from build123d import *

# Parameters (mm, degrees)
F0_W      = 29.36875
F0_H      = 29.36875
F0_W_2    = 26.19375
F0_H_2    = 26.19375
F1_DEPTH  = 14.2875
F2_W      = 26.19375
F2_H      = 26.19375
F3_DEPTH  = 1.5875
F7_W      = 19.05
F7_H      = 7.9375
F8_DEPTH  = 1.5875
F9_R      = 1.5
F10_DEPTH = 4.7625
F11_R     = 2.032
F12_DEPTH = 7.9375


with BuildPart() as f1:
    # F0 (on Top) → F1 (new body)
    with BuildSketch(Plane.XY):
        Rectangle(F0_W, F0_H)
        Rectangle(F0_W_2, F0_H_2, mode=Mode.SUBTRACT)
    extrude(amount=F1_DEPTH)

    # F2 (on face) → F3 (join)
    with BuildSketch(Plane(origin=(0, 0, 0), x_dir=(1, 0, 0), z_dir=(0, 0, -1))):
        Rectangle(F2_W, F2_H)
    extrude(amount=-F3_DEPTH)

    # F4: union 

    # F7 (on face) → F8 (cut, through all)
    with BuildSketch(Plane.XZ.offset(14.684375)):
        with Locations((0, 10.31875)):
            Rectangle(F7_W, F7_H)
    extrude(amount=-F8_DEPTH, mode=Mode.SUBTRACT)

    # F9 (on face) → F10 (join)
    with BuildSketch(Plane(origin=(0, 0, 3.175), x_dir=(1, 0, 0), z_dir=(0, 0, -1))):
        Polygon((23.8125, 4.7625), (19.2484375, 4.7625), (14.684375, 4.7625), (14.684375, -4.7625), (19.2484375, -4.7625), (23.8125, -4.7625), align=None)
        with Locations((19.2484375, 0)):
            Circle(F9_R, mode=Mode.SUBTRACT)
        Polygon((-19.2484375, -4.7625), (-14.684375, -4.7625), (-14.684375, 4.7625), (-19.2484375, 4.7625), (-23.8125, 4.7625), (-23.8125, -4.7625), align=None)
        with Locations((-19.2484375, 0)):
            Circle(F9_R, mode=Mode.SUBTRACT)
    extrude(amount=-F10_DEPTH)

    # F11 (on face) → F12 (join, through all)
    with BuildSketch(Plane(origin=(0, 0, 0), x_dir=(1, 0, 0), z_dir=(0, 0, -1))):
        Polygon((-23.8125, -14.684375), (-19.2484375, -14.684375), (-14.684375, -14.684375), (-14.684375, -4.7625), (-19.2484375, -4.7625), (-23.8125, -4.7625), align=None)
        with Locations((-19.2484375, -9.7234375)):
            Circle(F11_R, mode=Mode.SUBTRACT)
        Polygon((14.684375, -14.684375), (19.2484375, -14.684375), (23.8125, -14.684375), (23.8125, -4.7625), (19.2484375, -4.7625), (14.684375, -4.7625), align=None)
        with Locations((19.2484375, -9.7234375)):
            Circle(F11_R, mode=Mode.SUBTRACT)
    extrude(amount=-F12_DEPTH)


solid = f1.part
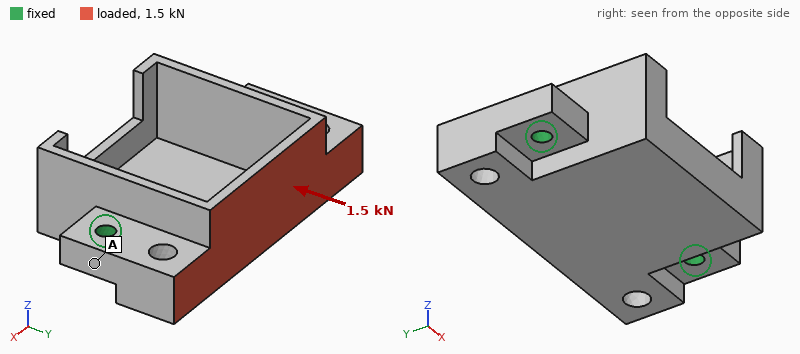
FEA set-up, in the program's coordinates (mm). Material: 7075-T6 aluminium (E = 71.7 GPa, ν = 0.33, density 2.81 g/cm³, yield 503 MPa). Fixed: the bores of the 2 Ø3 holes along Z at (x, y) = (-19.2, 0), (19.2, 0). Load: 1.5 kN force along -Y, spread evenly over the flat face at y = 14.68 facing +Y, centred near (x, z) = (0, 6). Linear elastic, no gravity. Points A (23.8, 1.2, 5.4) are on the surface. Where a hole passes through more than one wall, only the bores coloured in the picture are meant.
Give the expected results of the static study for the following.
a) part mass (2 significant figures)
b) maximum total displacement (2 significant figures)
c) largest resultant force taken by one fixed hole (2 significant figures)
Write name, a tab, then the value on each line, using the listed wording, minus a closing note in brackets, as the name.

part mass	15 g
maximum total displacement	0.18 mm
largest resultant force taken by one fixed hole	780 N
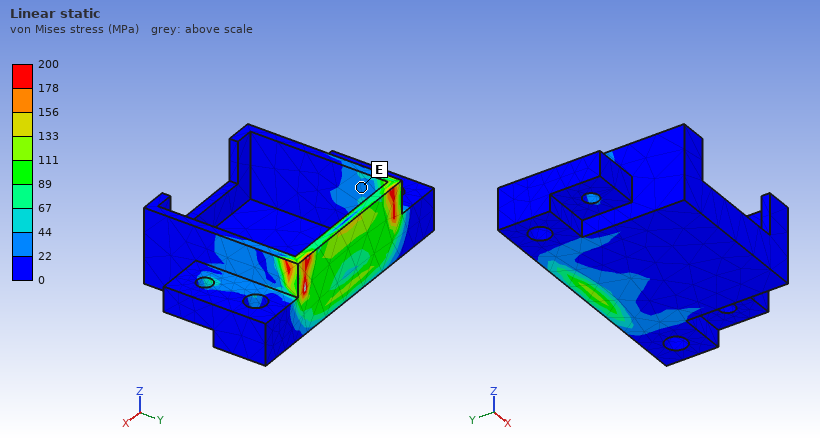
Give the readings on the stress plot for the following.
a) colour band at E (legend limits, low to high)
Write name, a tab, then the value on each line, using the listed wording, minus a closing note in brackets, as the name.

colour band at E	22 to 44 MPa
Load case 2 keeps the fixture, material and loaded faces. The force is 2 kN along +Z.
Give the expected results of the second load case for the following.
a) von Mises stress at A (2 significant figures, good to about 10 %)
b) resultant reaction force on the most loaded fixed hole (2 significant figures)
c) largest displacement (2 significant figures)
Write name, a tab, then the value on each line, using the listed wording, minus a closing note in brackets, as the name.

von Mises stress at A	87 MPa
resultant reaction force on the most loaded fixed hole	1.0 kN
largest displacement	0.18 mm
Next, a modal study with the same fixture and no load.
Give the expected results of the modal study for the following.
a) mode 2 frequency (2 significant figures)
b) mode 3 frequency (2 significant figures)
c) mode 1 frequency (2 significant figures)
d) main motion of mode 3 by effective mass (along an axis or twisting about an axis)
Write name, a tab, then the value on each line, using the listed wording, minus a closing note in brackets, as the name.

mode 2 frequency	11 kHz
mode 3 frequency	12 kHz
mode 1 frequency	8200 Hz
main motion of mode 3 by effective mass	along Z
